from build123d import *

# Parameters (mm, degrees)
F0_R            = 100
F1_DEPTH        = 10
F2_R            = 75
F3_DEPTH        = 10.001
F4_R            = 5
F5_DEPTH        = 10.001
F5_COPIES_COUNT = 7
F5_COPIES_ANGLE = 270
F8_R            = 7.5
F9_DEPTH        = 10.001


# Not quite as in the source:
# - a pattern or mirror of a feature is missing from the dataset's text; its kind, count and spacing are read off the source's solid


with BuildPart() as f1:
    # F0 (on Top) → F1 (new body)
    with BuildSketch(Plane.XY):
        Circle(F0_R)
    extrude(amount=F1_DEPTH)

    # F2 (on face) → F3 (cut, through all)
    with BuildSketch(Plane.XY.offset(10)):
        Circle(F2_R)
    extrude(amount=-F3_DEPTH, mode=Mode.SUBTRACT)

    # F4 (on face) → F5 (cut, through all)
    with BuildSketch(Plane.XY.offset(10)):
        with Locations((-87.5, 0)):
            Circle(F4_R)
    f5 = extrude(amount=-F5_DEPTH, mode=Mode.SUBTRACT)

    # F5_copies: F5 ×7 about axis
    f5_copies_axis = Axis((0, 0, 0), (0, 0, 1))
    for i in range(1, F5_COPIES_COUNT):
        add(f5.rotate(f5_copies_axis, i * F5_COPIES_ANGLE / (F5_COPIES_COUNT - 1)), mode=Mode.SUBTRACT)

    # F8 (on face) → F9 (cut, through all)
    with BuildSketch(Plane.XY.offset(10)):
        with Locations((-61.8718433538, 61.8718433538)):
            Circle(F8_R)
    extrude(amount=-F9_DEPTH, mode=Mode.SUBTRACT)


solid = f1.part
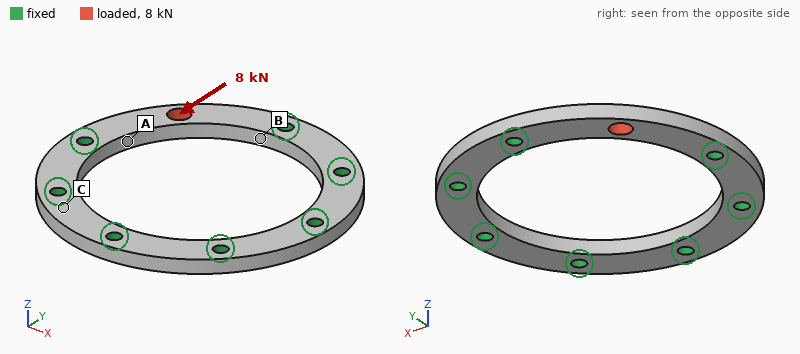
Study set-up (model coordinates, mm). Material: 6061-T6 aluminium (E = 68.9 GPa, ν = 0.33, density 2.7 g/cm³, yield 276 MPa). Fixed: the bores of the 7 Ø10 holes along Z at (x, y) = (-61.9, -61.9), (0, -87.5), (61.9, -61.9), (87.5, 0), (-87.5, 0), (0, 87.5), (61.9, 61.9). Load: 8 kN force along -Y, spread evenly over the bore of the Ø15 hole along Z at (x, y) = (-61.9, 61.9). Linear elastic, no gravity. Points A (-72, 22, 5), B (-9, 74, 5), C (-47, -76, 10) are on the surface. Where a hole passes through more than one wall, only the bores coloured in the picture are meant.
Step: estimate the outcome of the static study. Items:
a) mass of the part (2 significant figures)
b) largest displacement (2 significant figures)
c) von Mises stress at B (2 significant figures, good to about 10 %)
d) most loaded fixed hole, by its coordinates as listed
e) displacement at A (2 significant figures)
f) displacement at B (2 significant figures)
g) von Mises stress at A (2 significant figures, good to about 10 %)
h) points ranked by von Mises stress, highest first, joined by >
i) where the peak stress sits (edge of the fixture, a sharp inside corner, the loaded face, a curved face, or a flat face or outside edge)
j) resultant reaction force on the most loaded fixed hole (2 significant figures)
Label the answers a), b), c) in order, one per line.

a) 350 g
b) 70 µm
c) 41 MPa
d) (-87.5, 0)
e) 19 µm
f) 12 µm
g) 60 MPa
h) A > B > C
i) the loaded face
j) 7.2 kN
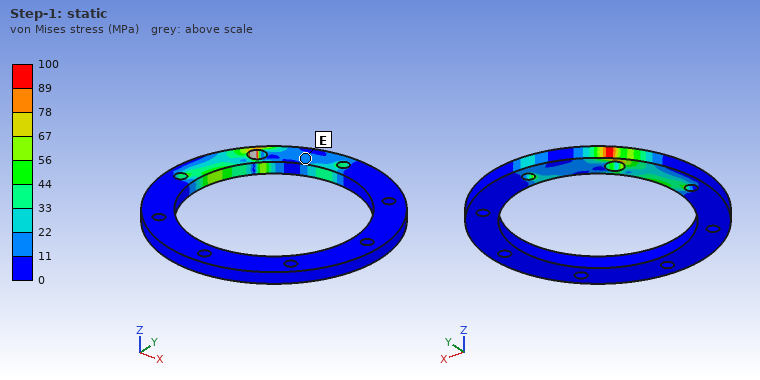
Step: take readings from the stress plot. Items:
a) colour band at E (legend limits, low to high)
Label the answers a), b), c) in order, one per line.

a) 11 to 22 MPa
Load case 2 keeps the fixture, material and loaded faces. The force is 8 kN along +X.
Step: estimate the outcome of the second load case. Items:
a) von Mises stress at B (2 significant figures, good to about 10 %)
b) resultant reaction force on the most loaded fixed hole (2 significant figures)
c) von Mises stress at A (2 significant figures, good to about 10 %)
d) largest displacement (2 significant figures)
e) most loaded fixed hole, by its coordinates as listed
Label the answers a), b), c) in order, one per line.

a) 42 MPa
b) 7.2 kN
c) 22 MPa
d) 70 µm
e) (0, 87.5)
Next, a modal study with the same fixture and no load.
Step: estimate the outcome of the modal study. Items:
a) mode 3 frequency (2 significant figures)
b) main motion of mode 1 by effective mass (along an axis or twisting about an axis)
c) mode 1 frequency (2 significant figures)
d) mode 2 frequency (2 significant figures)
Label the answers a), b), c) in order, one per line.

a) 8700 Hz
b) along Z
c) 2700 Hz
d) 6900 Hz
